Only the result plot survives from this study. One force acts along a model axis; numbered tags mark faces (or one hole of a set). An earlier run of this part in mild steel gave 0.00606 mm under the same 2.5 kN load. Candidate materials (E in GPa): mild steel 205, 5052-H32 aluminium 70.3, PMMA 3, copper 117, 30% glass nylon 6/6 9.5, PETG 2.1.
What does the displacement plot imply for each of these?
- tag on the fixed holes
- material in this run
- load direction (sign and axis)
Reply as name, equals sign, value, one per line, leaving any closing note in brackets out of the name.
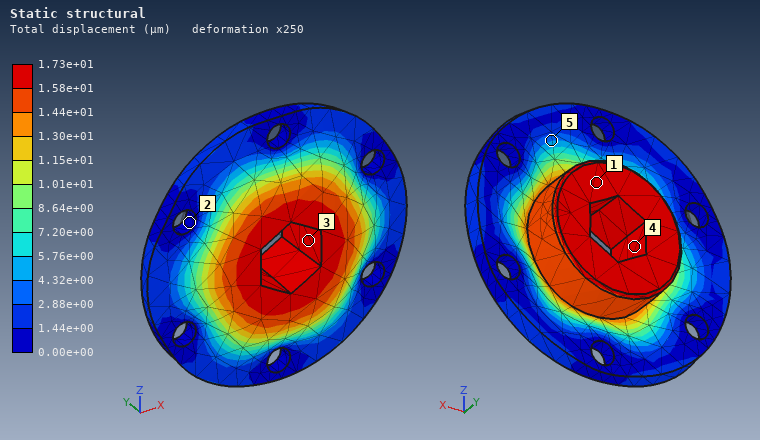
tag on the fixed holes = 2
material in this run = 5052-H32 aluminium
load direction = -Y
